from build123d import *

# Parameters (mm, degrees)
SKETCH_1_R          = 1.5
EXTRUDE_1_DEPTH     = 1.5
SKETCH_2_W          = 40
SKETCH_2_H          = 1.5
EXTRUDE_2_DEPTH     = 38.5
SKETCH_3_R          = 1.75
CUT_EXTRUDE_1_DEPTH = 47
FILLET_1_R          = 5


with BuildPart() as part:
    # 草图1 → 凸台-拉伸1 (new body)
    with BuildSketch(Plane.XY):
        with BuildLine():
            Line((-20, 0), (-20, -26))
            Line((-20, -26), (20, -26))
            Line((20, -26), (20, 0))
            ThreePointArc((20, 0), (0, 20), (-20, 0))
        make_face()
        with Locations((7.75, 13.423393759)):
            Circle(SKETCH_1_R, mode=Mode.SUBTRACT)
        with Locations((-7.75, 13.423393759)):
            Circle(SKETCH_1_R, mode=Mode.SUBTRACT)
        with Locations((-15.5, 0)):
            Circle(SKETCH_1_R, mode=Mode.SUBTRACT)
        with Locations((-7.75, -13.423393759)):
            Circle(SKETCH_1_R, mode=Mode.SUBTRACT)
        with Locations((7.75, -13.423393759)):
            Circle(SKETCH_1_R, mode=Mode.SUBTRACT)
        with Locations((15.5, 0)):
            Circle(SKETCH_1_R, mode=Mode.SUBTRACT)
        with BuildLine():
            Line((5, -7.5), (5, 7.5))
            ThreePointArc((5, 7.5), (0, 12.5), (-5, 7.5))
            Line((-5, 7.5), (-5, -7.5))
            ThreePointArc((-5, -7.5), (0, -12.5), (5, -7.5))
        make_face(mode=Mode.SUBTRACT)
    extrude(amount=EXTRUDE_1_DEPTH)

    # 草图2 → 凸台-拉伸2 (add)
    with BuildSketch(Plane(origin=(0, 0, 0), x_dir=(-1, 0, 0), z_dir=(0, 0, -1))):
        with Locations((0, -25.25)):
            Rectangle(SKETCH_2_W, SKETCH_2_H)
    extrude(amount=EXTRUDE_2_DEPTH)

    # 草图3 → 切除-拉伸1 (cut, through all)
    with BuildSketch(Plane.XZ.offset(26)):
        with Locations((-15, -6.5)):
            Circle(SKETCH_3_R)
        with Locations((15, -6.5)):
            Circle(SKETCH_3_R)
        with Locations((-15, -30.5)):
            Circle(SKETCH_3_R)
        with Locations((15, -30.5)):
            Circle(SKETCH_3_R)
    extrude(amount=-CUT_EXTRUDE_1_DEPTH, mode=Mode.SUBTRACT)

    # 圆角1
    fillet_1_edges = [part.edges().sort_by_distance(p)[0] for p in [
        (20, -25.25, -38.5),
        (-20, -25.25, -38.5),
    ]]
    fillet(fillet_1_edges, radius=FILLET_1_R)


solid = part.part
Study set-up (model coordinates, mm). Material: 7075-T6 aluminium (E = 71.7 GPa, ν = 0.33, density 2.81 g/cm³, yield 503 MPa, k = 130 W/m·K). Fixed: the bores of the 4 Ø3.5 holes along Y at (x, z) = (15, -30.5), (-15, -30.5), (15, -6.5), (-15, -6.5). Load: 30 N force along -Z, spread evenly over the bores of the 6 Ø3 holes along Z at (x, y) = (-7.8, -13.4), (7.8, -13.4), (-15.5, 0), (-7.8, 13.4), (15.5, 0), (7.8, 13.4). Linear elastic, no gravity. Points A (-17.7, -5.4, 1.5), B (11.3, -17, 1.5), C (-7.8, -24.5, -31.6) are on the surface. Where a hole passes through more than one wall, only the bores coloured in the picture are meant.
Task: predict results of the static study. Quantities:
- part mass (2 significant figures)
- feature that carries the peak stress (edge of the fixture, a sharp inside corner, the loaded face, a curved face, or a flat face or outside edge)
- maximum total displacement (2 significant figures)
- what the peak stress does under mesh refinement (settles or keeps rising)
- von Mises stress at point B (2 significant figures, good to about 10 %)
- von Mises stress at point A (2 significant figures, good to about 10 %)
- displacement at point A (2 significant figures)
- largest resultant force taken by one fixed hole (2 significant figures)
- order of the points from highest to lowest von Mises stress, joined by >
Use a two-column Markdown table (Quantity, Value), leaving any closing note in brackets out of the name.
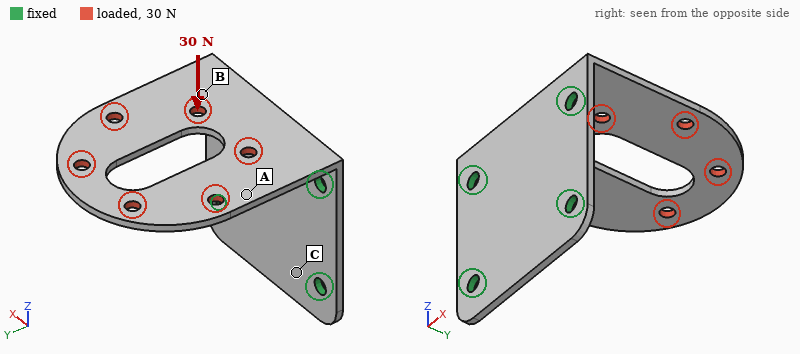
| Quantity | Value |
|---|---|
| part mass | 12 g |
| feature that carries the peak stress | edge of the fixture |
| maximum total displacement | 0.78 mm |
| what the peak stress does under mesh refinement | keeps rising |
| von Mises stress at point B | 33 MPa |
| von Mises stress at point A | 21 MPa |
| displacement at point A | 0.25 mm |
| largest resultant force taken by one fixed hole | 10 N |
| order of the points from highest to lowest von Mises stress, joined by > | B > A > C |
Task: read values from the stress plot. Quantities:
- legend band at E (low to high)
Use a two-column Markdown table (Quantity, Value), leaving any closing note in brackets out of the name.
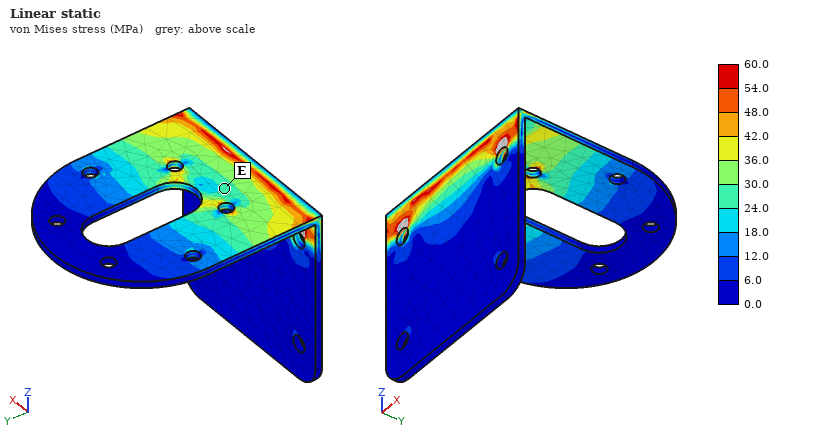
| Quantity | Value |
|---|---|
| legend band at E | 24.0 to 30.0 MPa |
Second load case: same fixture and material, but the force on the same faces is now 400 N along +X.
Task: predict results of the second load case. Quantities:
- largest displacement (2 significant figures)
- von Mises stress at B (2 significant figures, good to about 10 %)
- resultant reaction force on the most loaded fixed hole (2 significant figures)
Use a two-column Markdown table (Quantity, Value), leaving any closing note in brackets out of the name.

| Quantity | Value |
|---|---|
| largest displacement | 0.30 mm |
| von Mises stress at B | 26 MPa |
| resultant reaction force on the most loaded fixed hole | 390 N |
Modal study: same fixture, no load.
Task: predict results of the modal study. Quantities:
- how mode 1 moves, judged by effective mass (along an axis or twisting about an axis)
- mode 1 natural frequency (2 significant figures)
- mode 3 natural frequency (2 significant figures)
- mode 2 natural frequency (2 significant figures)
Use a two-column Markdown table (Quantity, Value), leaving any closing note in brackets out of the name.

| Quantity | Value |
|---|---|
| how mode 1 moves, judged by effective mass | along Z |
| mode 1 natural frequency | 610 Hz |
| mode 3 natural frequency | 3200 Hz |
| mode 2 natural frequency | 1700 Hz |
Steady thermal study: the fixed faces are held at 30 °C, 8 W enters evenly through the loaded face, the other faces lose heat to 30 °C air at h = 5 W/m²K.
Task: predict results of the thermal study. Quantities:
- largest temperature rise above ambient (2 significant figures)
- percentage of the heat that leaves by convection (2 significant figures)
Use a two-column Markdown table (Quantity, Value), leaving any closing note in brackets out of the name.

| Quantity | Value |
|---|---|
| largest temperature rise above ambient | 42 K |
| percentage of the heat that leaves by convection | 5.4 % |
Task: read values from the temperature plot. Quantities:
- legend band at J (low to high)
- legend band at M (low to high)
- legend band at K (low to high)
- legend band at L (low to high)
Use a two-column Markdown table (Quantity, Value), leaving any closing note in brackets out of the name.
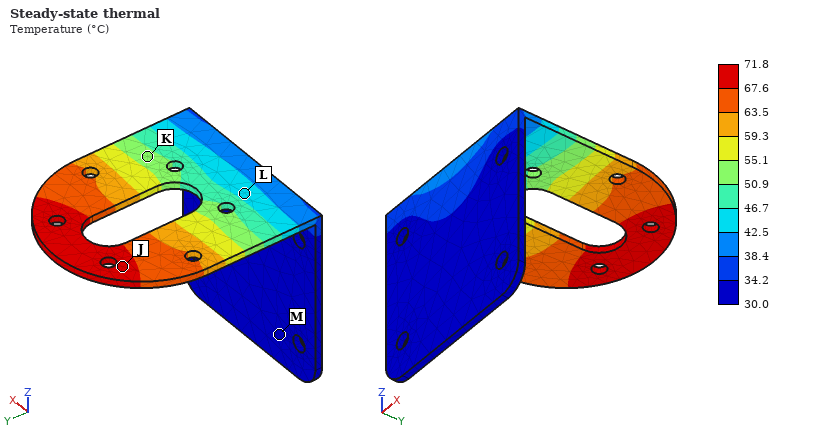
| Quantity | Value |
|---|---|
| legend band at J | 67.6 to 71.8 °C |
| legend band at M | 30.0 to 34.2 °C |
| legend band at K | 50.9 to 55.1 °C |
| legend band at L | 42.5 to 46.7 °C |
